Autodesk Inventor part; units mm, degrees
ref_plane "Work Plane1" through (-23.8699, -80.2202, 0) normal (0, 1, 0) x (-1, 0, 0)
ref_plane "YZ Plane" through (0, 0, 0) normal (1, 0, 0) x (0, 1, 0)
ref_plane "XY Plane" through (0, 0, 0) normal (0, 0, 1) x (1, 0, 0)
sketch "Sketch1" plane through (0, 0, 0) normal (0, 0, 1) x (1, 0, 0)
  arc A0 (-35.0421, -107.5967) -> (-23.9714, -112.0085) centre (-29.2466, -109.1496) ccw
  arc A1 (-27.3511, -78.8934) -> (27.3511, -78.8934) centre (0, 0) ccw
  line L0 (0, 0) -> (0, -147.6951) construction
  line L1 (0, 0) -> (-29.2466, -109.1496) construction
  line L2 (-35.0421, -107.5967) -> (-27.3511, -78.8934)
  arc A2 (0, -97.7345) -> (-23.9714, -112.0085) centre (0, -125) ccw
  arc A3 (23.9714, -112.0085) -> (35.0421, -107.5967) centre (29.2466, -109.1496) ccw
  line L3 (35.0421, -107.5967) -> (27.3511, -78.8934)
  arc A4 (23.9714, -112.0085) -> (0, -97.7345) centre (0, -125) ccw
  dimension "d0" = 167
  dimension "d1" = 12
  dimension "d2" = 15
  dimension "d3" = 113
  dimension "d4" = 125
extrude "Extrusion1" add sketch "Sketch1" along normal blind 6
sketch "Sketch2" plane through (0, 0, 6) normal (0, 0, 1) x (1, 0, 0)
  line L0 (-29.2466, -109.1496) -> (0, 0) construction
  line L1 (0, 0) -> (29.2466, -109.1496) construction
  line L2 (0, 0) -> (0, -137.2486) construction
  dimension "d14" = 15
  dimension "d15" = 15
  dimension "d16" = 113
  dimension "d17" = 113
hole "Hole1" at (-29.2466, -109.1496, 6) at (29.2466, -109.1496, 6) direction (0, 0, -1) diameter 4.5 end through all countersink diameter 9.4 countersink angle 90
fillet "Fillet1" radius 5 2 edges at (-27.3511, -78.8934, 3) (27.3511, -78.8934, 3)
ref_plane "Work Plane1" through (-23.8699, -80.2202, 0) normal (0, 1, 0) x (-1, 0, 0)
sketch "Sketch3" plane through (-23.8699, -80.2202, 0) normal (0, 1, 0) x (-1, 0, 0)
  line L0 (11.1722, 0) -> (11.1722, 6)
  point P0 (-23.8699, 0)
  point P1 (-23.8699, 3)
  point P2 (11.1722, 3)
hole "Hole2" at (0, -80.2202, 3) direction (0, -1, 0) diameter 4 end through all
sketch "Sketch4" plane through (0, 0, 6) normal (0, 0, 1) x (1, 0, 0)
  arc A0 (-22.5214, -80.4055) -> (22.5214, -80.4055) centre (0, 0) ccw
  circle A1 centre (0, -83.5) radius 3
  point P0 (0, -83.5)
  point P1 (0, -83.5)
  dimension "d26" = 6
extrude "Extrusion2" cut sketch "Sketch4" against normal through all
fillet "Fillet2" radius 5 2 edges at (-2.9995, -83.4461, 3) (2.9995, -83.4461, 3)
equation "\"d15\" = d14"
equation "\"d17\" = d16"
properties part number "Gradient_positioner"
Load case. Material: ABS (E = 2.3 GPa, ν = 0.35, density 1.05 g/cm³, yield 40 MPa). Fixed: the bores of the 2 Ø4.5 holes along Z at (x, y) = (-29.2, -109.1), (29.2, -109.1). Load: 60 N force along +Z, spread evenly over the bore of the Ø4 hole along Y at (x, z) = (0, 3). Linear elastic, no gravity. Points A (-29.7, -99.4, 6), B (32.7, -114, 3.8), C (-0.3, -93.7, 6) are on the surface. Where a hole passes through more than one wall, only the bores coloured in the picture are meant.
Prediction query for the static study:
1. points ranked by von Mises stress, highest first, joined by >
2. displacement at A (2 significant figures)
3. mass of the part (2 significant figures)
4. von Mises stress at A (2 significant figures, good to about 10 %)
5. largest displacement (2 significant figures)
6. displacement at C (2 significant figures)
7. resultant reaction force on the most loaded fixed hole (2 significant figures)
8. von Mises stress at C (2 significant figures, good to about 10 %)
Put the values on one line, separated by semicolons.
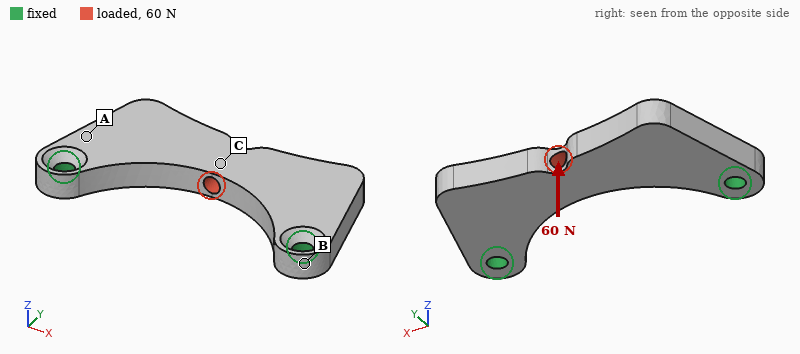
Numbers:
C > A > B; 0.069 mm; 8.7 g; 4.2 MPa; 0.44 mm; 0.33 mm; 30 N; 7.1 MPa
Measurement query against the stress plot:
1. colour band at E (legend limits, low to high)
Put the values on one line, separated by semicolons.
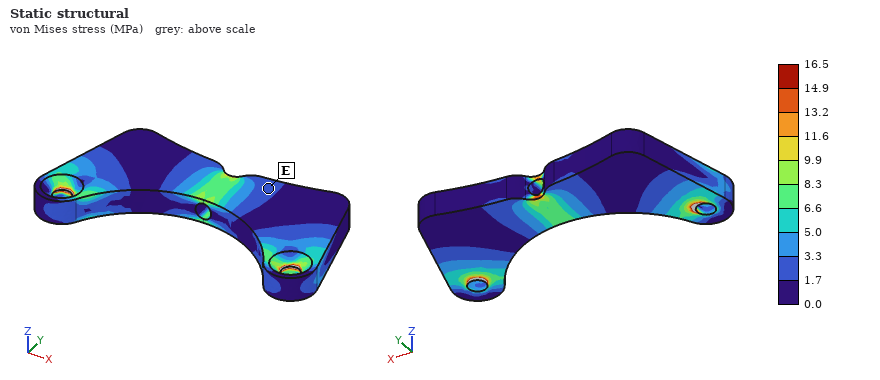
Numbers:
1.7 to 3.3 MPa
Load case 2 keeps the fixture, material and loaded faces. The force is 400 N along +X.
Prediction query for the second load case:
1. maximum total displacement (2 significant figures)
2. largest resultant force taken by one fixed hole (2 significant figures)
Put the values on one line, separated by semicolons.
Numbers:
97 µm; 220 N
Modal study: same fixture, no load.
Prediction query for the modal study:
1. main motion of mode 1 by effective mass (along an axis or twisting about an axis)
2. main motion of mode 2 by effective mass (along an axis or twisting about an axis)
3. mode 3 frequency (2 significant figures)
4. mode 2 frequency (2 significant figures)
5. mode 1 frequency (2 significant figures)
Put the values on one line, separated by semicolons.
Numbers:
along Z; twisting about Y; 3100 Hz; 2000 Hz; 980 Hz
